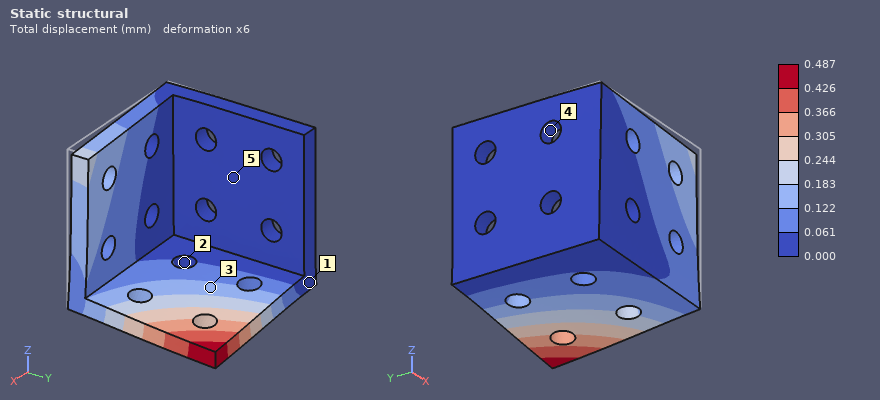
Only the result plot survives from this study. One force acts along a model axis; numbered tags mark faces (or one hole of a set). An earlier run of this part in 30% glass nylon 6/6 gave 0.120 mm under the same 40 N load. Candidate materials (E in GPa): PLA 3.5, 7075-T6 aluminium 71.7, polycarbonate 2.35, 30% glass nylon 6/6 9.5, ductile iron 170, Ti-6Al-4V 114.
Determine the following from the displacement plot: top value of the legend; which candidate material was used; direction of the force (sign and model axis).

0.487 mm
polycarbonate
-Z
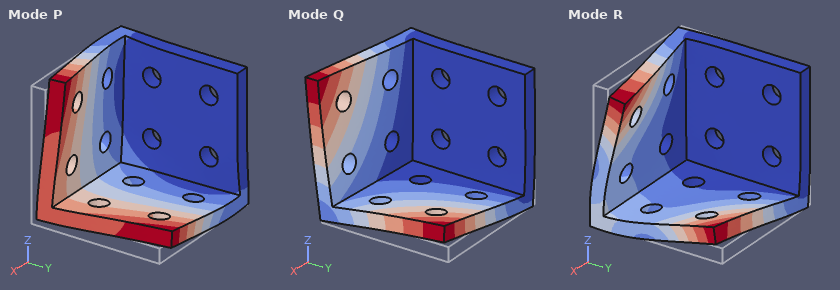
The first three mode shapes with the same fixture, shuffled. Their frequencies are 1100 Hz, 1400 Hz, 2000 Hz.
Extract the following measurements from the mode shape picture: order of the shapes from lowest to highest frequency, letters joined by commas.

Q, P, R
